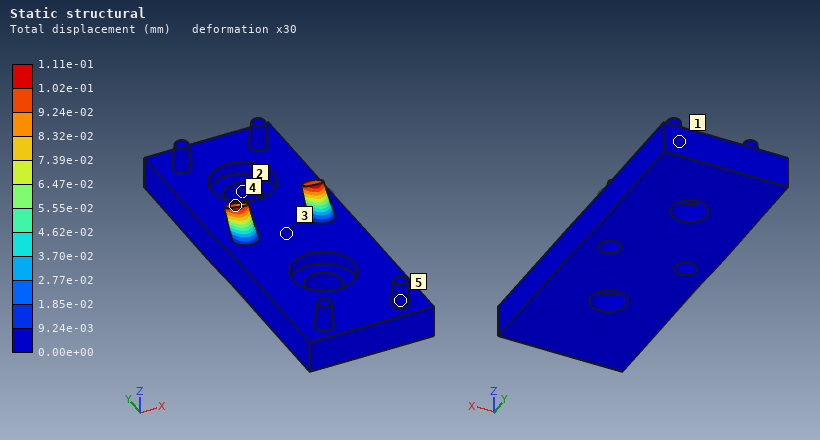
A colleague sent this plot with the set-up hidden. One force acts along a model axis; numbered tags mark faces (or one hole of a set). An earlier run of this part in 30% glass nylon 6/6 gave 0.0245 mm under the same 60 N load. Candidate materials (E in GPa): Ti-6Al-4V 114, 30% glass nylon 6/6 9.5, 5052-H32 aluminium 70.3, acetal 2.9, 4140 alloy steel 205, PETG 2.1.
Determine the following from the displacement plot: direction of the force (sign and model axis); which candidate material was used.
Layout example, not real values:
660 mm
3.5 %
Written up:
+Y
PETG
